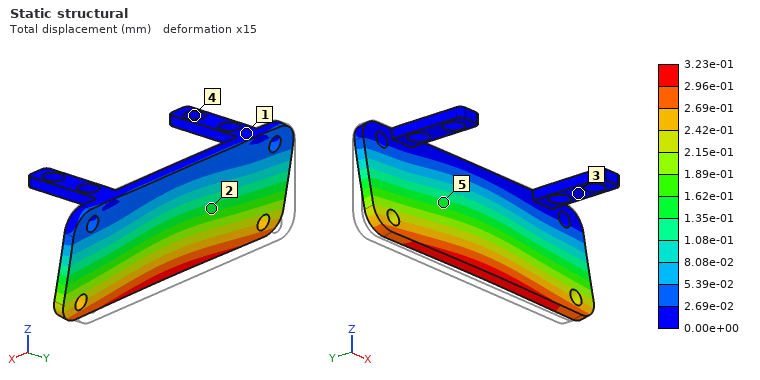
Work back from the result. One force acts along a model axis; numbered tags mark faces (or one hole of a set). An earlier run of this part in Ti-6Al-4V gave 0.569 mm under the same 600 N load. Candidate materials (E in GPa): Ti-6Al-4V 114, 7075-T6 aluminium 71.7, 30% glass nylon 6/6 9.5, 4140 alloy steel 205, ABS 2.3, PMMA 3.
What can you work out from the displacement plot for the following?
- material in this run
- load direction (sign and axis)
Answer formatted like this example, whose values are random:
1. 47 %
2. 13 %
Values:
1. 4140 alloy steel
2. -Y
